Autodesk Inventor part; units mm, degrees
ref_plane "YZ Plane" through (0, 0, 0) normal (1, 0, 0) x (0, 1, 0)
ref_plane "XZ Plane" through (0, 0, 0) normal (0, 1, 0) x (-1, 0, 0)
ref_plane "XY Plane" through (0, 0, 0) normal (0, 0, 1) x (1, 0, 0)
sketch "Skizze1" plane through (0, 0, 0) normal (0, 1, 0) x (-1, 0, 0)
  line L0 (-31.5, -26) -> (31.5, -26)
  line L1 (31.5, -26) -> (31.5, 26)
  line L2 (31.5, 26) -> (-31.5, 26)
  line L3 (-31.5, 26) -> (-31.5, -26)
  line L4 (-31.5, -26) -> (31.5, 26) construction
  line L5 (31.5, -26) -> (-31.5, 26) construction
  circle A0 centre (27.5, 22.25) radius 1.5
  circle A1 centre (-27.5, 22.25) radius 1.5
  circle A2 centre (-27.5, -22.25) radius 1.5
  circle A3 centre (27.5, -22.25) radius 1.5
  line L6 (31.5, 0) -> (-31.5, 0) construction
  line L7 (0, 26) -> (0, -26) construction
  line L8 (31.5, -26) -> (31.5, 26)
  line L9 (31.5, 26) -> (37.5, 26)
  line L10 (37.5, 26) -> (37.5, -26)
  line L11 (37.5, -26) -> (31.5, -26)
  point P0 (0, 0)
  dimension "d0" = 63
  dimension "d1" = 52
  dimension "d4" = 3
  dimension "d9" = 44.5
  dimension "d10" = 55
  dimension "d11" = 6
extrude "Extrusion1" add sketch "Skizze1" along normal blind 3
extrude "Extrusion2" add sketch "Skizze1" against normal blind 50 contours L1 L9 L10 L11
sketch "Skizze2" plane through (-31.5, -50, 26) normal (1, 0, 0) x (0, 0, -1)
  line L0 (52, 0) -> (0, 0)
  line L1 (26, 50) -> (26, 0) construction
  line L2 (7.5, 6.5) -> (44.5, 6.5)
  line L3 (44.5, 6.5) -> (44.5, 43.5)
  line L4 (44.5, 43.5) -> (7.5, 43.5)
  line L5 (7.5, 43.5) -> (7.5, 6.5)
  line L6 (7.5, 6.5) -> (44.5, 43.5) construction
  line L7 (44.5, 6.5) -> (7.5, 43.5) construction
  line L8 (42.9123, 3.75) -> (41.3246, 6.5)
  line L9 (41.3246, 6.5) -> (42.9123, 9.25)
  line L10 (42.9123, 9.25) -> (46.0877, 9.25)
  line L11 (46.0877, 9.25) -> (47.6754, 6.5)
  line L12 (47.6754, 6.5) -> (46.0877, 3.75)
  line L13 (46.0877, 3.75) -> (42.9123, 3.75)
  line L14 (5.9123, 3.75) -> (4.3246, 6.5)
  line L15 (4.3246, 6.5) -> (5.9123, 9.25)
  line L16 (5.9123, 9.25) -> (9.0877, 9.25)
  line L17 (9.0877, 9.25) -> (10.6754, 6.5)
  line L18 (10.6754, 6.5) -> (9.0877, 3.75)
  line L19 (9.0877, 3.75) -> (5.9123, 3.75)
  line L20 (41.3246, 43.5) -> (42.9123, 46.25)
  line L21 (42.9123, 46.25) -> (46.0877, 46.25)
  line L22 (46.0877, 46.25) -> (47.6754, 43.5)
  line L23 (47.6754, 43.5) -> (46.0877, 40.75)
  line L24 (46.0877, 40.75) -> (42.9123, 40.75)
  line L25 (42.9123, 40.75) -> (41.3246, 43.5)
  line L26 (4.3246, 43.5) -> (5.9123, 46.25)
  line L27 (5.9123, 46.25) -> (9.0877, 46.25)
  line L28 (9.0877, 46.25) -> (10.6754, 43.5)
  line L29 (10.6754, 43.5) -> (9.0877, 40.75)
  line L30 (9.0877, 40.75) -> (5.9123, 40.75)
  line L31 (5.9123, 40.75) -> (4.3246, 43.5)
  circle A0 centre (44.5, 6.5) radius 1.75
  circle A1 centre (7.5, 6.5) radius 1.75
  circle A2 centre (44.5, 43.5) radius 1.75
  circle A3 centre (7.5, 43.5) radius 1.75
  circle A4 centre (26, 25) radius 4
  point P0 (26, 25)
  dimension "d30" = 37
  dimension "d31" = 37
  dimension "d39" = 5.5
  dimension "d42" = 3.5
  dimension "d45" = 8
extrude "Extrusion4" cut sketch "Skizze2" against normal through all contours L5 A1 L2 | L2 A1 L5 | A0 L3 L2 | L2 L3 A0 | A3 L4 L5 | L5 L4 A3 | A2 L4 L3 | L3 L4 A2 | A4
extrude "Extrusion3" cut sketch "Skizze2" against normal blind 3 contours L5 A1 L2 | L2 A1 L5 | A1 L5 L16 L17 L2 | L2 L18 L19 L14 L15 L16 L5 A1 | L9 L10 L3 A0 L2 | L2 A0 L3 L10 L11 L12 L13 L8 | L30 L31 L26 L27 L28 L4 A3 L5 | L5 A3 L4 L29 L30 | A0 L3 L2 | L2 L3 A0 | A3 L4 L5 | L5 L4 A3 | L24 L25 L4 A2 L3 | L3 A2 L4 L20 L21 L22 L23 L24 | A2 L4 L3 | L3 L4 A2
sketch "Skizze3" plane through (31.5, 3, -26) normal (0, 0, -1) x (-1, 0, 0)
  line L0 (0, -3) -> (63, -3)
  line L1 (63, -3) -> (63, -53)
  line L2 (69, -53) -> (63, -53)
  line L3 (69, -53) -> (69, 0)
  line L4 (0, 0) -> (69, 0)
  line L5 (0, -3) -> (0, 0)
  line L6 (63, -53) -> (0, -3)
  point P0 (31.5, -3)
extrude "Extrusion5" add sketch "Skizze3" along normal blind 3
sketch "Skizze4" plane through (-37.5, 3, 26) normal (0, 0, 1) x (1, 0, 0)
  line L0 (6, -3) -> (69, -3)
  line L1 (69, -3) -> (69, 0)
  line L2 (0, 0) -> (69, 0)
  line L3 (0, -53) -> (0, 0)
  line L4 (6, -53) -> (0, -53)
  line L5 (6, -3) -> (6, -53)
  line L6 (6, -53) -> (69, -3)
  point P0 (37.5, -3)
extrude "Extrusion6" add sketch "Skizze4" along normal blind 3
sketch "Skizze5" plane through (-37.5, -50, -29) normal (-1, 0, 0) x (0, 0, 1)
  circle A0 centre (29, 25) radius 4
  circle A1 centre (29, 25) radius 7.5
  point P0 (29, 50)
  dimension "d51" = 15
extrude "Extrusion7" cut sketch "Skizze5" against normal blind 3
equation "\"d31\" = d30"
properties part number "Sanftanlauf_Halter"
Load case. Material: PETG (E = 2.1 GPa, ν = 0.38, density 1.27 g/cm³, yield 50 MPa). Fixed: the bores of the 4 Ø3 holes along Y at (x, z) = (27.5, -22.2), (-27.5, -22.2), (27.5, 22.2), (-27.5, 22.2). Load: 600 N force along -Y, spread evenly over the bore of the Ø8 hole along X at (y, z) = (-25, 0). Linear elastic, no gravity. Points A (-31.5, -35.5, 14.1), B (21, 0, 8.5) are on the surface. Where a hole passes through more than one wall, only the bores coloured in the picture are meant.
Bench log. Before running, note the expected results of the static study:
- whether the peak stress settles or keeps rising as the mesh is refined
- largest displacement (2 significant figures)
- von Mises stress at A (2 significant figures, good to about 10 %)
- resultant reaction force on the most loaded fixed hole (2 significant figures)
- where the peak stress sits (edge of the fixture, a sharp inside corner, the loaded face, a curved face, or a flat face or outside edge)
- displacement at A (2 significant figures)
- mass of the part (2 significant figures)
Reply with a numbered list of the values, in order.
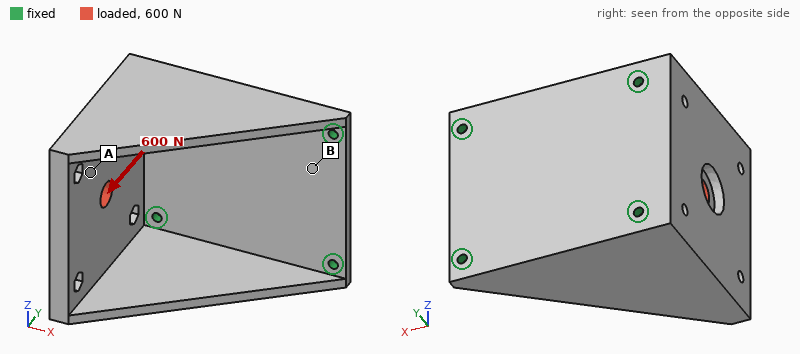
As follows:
1. keeps rising
2. 0.21 mm
3. 2.4 MPa
4. 330 N
5. edge of the fixture
6. 0.18 mm
7. 48 g
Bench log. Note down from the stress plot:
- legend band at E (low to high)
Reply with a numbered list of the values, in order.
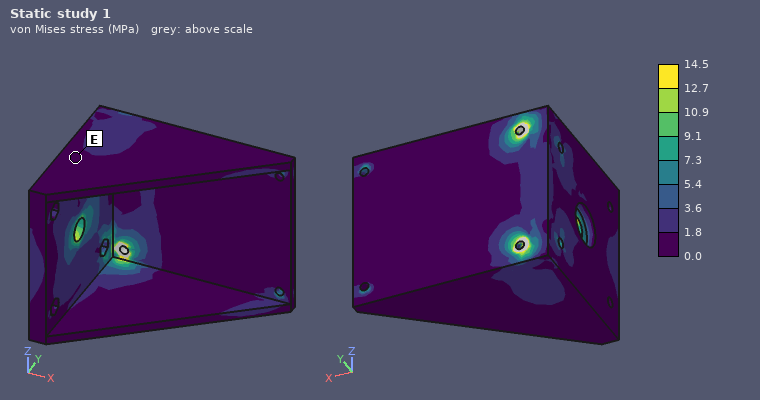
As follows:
1. 0.0 to 1.8 MPa
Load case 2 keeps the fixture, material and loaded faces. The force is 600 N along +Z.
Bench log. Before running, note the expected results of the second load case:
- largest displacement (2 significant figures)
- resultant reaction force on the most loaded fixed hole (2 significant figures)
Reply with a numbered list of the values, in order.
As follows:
1. 0.53 mm
2. 480 N
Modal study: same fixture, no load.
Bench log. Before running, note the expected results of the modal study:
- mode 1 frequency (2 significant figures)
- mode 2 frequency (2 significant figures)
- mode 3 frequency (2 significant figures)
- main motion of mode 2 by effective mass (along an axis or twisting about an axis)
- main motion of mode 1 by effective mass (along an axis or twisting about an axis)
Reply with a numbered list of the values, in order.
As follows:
1. 930 Hz
2. 1100 Hz
3. 1200 Hz
4. along Z
5. along X
